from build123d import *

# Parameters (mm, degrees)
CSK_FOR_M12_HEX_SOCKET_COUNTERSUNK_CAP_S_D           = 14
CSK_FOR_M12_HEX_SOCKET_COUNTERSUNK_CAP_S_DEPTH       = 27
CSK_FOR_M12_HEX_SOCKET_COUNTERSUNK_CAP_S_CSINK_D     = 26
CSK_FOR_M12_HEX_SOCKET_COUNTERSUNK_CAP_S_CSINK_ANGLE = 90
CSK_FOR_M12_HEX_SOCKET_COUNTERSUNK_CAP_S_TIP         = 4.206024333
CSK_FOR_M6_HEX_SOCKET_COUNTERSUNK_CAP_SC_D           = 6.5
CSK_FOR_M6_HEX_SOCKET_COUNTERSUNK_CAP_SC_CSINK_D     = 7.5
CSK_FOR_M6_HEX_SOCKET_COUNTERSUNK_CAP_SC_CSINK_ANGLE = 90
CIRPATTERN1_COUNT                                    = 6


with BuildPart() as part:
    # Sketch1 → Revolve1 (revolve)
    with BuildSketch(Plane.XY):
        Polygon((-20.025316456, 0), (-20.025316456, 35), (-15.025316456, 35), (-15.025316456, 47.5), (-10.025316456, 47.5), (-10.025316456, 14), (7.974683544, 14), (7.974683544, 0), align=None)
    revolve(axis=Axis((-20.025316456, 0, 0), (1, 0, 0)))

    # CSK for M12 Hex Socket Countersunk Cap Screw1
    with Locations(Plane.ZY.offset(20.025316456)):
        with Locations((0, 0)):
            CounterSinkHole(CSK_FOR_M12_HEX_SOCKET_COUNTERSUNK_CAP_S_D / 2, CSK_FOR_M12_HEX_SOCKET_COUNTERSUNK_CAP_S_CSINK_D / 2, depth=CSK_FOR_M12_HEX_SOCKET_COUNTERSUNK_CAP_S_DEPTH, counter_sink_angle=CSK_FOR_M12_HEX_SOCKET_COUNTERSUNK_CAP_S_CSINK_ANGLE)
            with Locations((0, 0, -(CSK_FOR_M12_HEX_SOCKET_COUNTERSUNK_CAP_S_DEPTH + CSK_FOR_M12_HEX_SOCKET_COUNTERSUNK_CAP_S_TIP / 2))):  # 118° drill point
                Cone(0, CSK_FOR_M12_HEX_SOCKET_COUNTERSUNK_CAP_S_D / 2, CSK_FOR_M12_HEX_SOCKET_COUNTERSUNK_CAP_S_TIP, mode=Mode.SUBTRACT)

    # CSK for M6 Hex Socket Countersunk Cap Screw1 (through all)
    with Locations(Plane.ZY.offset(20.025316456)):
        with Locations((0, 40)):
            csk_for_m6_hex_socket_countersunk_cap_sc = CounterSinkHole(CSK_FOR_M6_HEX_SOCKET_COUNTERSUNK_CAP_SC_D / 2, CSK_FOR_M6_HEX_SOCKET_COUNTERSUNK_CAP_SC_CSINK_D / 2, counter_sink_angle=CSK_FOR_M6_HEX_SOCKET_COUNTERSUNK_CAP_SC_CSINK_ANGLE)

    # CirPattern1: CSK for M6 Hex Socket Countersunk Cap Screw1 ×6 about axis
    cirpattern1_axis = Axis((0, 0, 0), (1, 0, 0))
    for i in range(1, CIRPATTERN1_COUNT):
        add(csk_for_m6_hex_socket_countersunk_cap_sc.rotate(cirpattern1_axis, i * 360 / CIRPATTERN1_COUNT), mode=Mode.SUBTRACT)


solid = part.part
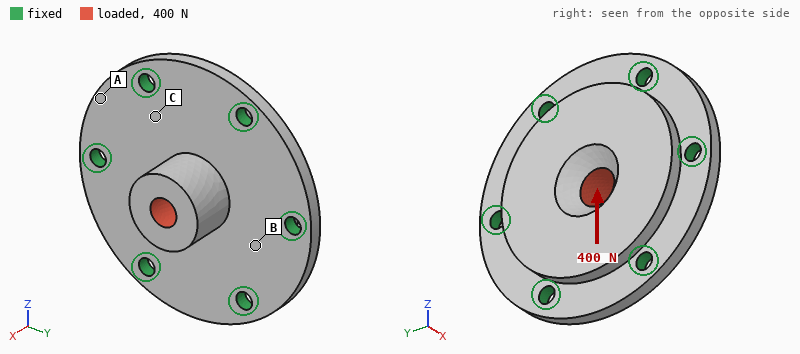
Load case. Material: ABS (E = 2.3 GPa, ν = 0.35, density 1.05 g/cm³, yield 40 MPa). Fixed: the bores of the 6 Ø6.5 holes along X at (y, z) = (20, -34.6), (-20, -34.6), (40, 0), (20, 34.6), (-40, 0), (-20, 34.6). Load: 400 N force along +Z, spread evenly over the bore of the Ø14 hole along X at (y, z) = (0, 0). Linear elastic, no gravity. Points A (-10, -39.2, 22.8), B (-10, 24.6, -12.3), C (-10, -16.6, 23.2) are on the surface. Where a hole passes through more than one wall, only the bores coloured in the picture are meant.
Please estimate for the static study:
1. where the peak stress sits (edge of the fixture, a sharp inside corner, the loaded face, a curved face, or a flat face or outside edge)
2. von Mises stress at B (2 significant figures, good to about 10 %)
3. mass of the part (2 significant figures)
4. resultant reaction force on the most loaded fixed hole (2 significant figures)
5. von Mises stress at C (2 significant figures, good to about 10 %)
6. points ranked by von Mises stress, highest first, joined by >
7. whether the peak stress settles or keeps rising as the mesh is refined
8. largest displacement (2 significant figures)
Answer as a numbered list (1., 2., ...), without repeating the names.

1. edge of the fixture
2. 0.78 MPa
3. 62 g
4. 84 N
5. 1.2 MPa
6. C > B > A
7. keeps rising
8. 65 µm
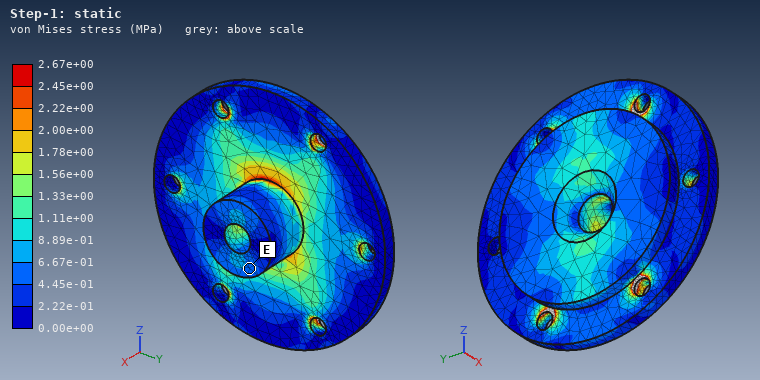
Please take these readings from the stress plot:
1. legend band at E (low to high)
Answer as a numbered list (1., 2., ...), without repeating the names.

1. 4.45e-01 to 6.67e-01 MPa
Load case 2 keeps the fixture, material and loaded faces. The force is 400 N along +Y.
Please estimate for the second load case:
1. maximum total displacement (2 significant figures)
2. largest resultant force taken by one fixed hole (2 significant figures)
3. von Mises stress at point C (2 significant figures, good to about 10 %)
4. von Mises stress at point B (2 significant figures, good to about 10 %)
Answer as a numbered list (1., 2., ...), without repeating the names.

1. 65 µm
2. 93 N
3. 0.71 MPa
4. 0.85 MPa
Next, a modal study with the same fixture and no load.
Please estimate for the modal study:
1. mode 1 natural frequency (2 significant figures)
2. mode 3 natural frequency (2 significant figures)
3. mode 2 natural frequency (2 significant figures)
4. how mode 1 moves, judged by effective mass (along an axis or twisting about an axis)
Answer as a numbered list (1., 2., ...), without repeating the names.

1. 2400 Hz
2. 3600 Hz
3. 3600 Hz
4. along X
